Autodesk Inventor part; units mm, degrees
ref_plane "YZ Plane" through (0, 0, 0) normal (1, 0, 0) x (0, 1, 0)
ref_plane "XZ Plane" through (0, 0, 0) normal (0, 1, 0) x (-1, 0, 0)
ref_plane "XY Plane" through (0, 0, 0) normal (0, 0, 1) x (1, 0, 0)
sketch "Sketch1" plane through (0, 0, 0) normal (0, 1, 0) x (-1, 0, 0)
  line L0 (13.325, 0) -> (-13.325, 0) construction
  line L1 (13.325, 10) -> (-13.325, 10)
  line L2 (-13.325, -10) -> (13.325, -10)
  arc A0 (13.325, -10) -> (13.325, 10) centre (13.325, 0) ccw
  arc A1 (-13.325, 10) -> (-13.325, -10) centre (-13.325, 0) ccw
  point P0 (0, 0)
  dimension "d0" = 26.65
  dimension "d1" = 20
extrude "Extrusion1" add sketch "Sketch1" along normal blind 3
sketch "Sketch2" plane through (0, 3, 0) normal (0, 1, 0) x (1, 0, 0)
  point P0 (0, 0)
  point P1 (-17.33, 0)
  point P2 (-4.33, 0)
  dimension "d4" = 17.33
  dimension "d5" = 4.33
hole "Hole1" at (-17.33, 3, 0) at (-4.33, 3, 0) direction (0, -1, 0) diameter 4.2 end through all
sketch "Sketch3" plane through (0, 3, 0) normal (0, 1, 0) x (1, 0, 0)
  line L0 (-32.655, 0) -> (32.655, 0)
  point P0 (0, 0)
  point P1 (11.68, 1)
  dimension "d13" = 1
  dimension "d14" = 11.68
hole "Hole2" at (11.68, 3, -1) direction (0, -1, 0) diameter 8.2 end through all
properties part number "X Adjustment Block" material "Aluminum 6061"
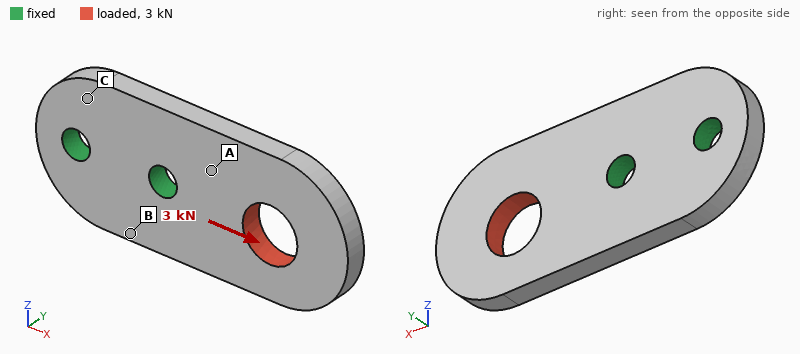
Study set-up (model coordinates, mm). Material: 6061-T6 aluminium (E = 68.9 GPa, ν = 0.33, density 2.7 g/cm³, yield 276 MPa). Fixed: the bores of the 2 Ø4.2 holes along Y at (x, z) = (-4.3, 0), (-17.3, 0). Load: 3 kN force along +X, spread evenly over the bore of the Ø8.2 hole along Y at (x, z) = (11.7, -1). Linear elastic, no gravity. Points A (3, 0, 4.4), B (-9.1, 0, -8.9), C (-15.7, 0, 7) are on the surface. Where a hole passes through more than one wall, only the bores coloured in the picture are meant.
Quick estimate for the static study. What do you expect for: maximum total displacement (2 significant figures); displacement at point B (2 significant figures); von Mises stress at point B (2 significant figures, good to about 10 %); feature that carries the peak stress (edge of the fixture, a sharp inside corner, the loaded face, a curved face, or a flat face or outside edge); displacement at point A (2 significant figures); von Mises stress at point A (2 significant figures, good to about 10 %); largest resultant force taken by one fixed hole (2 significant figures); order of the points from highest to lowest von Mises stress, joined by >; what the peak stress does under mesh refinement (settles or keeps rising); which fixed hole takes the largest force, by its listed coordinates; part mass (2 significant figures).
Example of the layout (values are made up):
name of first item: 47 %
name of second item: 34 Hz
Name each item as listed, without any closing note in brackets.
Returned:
maximum total displacement: 28 µm
displacement at point B: 4.6 µm
von Mises stress at point B: 30 MPa
feature that carries the peak stress: edge of the fixture
displacement at point A: 6.1 µm
von Mises stress at point A: 55 MPa
largest resultant force taken by one fixed hole: 2.4 kN
order of the points from highest to lowest von Mises stress, joined by >: A > B > C
what the peak stress does under mesh refinement: keeps rising
which fixed hole takes the largest force, by its listed coordinates: (-4.3, 0)
part mass: 6.2 g
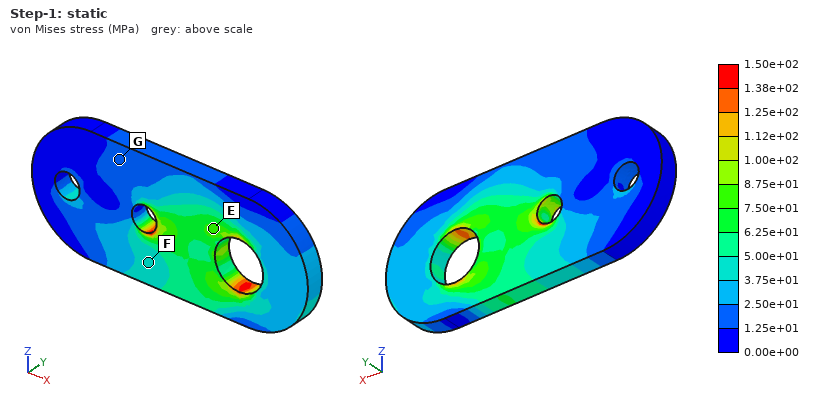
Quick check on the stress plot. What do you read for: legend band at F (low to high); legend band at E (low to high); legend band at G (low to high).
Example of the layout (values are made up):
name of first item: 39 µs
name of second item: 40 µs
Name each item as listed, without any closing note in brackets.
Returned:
legend band at F: 3.75e+01 to 5.00e+01 MPa
legend band at E: 7.50e+01 to 8.75e+01 MPa
legend band at G: 1.25e+01 to 2.50e+01 MPa
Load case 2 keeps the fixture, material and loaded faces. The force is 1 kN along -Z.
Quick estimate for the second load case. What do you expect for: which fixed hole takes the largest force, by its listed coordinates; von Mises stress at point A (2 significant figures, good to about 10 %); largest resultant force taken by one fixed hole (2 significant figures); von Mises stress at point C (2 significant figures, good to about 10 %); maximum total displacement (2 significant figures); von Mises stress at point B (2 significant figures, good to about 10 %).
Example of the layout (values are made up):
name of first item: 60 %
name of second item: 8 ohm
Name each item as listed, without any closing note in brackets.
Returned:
which fixed hole takes the largest force, by its listed coordinates: (-4.3, 0)
von Mises stress at point A: 32 MPa
largest resultant force taken by one fixed hole: 1.8 kN
von Mises stress at point C: 18 MPa
maximum total displacement: 68 µm
von Mises stress at point B: 41 MPa
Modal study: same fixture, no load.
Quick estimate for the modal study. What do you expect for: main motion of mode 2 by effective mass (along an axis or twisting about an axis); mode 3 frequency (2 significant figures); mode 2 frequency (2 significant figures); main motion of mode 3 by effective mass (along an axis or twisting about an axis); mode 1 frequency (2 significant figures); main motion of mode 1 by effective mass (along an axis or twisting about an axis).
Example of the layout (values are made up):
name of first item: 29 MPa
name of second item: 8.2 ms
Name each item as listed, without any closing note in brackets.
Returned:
main motion of mode 2 by effective mass: twisting about X
mode 3 frequency: 13 kHz
mode 2 frequency: 9400 Hz
main motion of mode 3 by effective mass: along Z
mode 1 frequency: 3900 Hz
main motion of mode 1 by effective mass: along Y
